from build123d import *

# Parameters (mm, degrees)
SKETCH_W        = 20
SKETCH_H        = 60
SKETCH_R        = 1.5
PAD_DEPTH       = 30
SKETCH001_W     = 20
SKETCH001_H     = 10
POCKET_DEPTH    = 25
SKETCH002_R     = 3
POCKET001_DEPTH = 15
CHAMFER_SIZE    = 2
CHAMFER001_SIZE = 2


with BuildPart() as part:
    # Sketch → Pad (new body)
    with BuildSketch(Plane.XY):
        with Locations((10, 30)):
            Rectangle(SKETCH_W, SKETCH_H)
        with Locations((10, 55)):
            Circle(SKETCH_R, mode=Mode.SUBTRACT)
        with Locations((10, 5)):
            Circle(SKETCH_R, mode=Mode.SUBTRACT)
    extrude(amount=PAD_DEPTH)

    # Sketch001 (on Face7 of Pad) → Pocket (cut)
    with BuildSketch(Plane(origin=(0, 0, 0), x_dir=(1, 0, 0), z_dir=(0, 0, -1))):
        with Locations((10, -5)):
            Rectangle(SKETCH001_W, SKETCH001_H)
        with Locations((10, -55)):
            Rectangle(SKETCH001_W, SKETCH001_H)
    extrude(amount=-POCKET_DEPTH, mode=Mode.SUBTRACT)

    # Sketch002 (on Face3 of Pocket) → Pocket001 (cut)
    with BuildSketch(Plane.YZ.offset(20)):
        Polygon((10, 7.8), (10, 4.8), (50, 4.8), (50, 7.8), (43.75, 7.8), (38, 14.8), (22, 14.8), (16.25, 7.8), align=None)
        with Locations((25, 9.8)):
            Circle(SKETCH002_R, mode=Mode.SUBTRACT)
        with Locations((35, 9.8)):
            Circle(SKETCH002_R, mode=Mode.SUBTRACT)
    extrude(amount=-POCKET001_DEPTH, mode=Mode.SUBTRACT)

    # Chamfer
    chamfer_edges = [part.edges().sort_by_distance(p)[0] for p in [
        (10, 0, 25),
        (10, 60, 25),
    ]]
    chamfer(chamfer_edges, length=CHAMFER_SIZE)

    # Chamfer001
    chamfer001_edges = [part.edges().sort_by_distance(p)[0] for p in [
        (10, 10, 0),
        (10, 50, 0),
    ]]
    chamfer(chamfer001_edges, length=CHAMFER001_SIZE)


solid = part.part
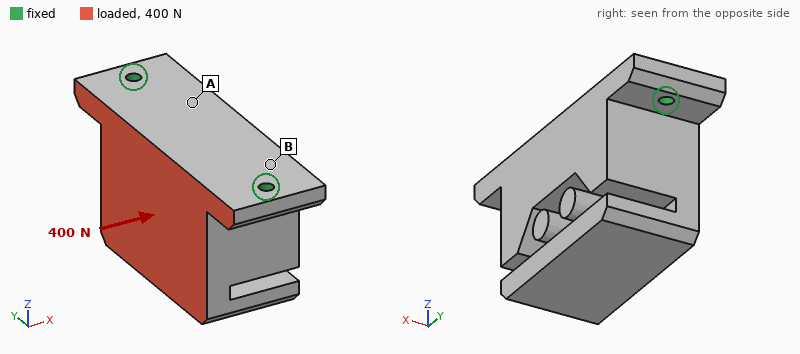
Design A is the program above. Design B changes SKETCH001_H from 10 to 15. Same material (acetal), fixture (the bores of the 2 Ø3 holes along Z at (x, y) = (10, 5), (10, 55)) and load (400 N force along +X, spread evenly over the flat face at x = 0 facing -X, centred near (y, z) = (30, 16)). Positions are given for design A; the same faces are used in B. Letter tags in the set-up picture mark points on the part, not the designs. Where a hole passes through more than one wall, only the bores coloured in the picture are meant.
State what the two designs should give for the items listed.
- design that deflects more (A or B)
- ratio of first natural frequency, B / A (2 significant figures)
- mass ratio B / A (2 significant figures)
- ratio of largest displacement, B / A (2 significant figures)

B
0.96
0.90
1.2
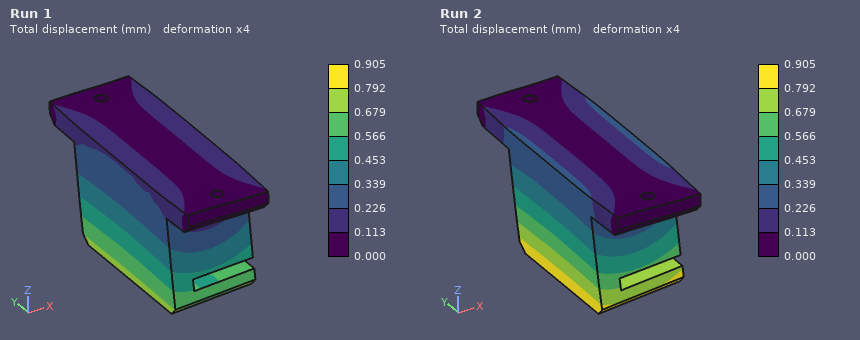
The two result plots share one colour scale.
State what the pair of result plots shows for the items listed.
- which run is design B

Run 2
